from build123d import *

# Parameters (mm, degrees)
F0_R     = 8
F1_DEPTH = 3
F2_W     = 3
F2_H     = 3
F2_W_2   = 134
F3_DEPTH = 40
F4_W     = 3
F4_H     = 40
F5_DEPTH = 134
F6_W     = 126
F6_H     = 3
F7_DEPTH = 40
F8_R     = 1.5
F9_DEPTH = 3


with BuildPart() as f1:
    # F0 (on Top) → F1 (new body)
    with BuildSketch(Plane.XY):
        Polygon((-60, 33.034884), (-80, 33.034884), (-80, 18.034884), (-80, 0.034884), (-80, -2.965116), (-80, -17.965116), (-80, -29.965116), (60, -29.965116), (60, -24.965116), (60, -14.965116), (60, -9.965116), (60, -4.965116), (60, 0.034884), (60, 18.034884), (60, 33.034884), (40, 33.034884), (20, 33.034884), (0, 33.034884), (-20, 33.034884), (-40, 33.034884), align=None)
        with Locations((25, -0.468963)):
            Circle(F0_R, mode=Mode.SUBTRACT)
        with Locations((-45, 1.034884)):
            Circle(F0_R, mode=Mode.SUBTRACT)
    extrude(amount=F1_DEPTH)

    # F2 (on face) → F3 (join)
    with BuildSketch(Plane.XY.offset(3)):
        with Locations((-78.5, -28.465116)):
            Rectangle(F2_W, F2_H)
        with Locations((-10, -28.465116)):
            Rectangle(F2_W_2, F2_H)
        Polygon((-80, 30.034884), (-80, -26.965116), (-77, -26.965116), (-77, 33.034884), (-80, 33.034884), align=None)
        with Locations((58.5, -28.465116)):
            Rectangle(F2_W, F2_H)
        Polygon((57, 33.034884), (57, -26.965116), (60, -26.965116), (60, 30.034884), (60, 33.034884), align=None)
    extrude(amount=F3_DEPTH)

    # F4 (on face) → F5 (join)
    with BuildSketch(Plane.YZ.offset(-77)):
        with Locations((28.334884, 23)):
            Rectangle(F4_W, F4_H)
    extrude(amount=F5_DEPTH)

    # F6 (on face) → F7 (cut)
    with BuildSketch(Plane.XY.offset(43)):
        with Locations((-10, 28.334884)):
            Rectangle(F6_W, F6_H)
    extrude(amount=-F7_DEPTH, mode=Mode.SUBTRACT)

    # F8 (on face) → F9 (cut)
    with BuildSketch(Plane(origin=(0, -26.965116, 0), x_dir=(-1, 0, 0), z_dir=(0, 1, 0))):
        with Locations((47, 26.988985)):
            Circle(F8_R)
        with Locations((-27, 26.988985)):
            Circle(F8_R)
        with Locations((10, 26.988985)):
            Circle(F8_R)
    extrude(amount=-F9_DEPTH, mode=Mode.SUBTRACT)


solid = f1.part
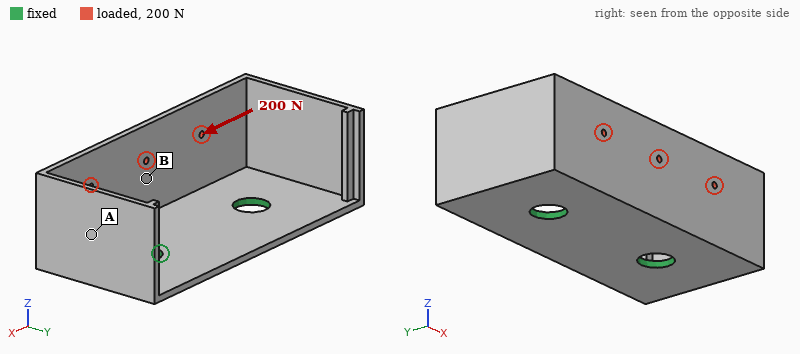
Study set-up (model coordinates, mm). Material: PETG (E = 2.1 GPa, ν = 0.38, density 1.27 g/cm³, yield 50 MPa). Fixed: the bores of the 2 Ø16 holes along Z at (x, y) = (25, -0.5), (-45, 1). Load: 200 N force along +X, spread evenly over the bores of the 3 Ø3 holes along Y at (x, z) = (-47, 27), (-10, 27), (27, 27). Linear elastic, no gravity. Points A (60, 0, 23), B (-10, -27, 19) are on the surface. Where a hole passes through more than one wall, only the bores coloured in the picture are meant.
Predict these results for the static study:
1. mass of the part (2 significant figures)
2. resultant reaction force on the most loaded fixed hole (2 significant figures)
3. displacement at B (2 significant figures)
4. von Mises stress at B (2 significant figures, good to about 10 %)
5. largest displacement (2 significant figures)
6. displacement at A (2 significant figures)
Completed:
73 g
130 N
0.32 mm
3.4 MPa
1.7 mm
0.65 mm
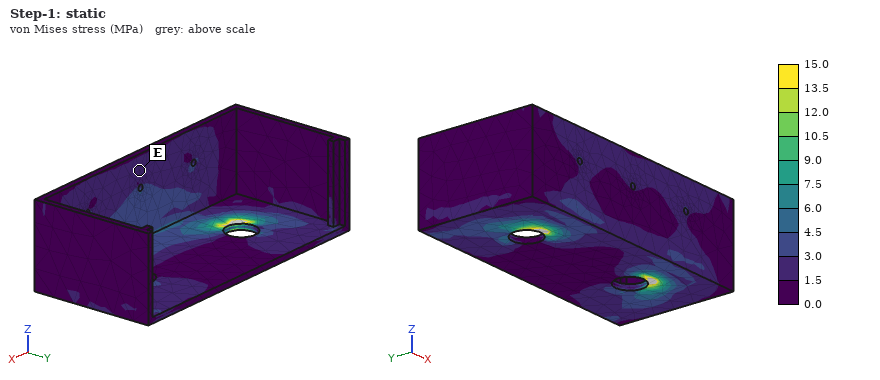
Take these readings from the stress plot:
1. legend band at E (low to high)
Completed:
1.5 to 3.0 MPa
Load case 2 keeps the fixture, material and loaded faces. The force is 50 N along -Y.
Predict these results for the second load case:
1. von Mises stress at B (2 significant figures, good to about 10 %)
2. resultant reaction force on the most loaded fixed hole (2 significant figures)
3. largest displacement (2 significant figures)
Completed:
1.6 MPa
26 N
1.8 mm
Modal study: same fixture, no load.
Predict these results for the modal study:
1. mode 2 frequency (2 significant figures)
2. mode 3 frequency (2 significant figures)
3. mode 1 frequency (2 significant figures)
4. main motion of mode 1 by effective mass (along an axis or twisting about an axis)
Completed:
240 Hz
290 Hz
200 Hz
along Y
